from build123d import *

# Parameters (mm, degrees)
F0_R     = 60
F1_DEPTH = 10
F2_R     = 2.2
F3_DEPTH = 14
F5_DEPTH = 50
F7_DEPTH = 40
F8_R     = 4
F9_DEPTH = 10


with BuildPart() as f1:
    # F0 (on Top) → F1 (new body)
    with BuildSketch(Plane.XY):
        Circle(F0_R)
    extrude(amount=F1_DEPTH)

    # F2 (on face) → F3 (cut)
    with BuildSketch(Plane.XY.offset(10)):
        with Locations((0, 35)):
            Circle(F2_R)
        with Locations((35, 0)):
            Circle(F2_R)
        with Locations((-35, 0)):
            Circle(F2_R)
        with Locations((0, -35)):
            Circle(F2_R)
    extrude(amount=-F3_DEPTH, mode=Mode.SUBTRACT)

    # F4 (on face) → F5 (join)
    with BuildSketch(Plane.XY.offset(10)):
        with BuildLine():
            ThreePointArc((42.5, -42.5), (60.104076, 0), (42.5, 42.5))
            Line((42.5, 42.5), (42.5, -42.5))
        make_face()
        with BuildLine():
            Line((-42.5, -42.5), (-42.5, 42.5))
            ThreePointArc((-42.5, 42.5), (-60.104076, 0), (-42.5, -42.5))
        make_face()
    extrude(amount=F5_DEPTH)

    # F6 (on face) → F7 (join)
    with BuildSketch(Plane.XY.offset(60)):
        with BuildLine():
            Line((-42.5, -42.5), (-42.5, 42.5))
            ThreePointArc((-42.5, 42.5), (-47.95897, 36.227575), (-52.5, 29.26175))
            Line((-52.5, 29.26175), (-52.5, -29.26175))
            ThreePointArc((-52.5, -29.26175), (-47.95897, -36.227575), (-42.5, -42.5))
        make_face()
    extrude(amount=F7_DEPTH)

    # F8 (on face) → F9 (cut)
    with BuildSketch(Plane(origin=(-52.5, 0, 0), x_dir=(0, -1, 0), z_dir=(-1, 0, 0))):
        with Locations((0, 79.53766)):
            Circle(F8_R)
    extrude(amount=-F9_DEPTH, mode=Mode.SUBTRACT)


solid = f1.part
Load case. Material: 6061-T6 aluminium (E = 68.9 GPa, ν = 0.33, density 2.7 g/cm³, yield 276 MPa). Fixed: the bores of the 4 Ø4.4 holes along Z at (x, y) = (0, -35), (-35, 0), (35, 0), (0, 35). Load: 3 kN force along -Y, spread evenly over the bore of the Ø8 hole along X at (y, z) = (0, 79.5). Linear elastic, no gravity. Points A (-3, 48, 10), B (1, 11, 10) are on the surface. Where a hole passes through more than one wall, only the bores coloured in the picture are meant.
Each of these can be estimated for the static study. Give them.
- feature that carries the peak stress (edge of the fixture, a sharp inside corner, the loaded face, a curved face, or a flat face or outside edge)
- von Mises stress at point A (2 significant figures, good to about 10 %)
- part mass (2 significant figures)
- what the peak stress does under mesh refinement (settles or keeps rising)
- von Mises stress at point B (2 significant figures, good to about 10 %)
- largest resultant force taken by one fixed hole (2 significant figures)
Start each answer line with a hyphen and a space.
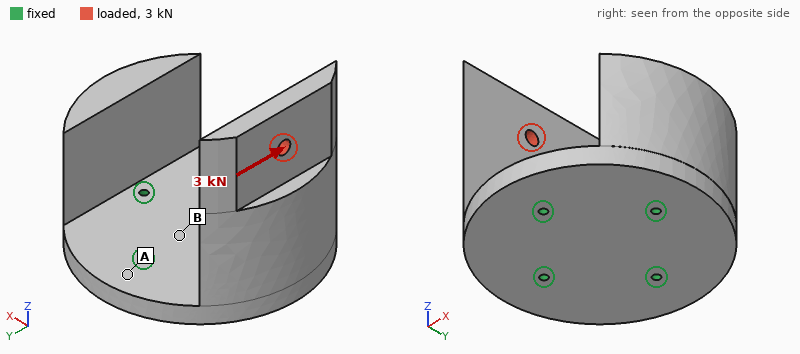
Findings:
- edge of the fixture
- 38 MPa
- 660 g
- keeps rising
- 16 MPa
- 2.5 kN
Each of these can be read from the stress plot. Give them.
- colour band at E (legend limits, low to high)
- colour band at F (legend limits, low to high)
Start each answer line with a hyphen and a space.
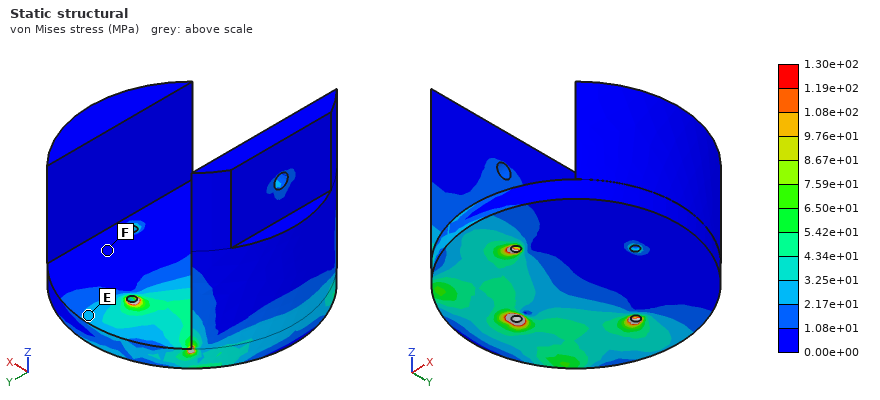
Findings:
- 2.17e+01 to 3.25e+01 MPa
- 0.00e+00 to 1.08e+01 MPa
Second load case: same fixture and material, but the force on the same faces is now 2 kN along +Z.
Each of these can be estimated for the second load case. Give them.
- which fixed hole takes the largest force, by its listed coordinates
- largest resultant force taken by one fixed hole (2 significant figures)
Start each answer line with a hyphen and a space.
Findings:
- (-35, 0)
- 2.2 kN
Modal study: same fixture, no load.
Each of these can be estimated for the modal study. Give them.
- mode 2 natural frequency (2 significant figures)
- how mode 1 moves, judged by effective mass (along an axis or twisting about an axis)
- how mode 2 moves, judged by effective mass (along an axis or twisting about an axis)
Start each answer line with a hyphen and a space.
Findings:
- 1400 Hz
- along X
- along Y
